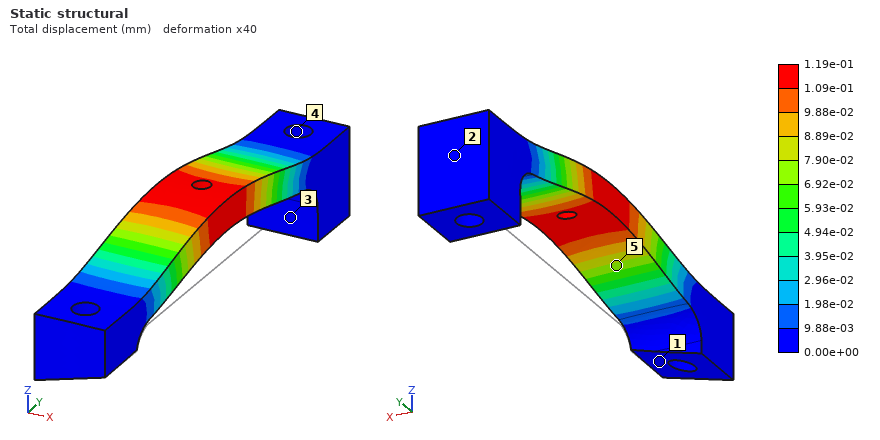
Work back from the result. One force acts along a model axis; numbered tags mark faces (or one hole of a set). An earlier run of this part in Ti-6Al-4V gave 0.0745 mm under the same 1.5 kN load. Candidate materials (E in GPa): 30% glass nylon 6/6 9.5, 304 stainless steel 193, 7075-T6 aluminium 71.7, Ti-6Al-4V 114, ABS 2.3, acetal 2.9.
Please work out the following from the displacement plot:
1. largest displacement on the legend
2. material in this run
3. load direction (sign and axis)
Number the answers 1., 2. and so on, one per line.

1. 1.19e-01 mm
2. 7075-T6 aluminium
3. +Z
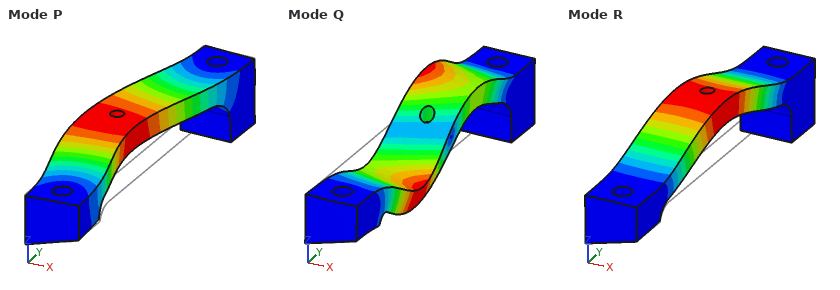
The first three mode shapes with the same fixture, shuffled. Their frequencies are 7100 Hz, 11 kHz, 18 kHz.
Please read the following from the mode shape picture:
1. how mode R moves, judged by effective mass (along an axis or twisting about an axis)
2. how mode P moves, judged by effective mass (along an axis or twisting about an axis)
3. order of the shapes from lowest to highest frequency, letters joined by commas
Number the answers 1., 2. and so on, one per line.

1. along Z
2. along X
3. R, P, Q
